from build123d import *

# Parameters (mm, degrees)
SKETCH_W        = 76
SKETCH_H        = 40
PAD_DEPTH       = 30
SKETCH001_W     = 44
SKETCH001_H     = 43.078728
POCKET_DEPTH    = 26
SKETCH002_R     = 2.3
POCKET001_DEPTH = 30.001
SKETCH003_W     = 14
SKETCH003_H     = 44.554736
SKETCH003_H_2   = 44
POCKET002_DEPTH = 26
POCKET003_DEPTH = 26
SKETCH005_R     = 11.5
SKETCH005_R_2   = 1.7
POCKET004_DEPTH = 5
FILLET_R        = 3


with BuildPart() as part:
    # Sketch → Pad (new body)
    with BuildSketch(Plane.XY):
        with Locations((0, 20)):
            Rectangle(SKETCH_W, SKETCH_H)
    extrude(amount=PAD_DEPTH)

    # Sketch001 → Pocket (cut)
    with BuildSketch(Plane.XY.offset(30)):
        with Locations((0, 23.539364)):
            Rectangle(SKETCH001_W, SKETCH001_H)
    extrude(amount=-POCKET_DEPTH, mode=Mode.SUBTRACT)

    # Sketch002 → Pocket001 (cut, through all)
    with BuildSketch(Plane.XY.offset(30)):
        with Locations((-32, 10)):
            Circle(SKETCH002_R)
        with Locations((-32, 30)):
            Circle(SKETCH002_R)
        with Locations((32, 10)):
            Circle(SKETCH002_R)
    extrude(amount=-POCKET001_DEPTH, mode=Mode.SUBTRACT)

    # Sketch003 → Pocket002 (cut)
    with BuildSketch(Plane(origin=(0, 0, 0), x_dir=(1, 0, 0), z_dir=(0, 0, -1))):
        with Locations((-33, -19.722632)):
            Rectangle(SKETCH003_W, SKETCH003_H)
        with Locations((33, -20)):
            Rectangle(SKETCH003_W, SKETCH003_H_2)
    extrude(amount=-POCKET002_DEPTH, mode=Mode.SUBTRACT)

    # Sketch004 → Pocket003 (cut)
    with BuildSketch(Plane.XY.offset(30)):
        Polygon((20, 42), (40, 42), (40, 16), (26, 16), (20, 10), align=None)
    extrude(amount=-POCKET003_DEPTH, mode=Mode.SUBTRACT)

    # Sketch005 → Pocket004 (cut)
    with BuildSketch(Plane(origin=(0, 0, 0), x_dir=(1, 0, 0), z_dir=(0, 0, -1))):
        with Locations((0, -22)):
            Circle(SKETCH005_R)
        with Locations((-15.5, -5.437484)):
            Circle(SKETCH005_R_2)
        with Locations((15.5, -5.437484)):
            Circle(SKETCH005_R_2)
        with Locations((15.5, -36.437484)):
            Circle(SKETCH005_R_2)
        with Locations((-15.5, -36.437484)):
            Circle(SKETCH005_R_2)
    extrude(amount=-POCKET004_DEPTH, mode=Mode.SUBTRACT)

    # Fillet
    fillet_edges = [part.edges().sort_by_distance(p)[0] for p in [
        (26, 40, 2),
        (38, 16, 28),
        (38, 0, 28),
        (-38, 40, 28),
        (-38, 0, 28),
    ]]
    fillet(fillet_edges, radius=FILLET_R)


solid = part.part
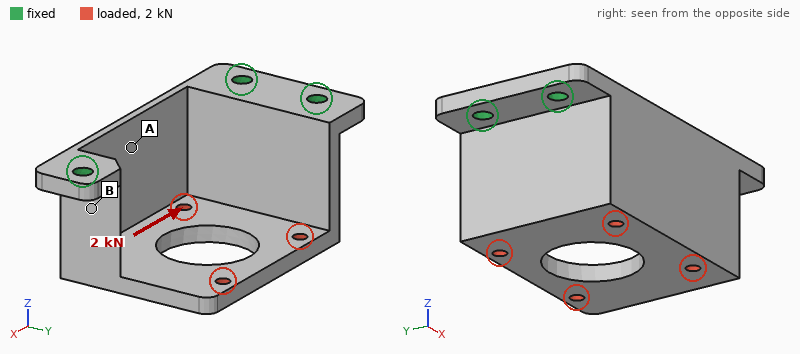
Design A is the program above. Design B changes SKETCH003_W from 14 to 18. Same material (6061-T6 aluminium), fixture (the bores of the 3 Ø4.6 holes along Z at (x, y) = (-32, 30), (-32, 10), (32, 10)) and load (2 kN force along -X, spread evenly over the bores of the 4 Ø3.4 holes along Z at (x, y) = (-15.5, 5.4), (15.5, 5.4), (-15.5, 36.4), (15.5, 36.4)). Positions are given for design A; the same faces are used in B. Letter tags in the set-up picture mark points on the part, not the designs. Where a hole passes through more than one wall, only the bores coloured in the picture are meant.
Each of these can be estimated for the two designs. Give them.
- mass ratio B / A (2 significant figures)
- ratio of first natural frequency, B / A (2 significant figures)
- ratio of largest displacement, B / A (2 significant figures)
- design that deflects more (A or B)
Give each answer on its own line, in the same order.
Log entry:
0.82
0.76
2.1
B
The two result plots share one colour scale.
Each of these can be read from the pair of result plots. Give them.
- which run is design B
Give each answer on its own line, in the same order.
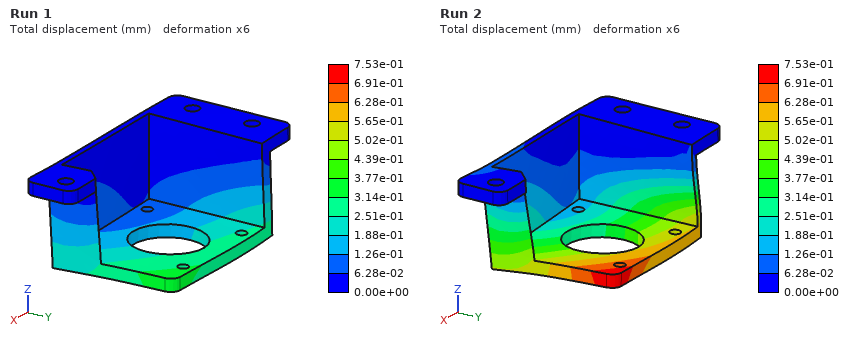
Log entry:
Run 2
